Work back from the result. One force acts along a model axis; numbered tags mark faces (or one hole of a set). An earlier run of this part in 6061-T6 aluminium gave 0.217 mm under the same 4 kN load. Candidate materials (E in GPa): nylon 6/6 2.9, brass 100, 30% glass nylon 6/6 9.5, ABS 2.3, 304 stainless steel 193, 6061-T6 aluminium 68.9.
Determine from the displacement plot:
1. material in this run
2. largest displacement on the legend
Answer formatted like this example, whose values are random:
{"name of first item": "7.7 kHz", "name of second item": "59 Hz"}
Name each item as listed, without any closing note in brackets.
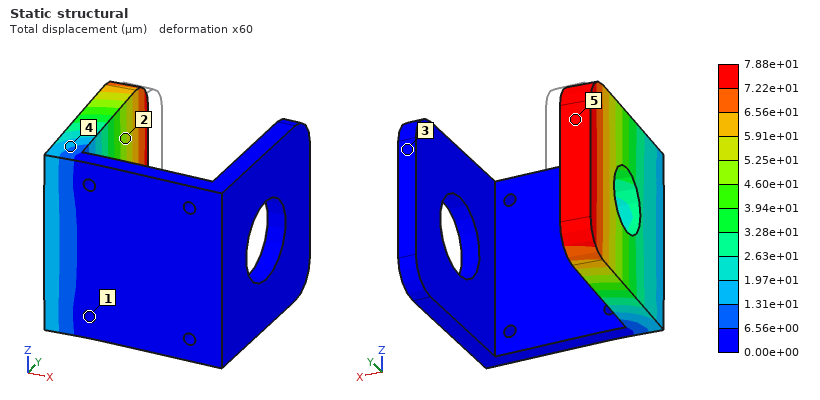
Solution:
{"material in this run": "304 stainless steel", "largest displacement on the legend": "7.88e+01 µm"}
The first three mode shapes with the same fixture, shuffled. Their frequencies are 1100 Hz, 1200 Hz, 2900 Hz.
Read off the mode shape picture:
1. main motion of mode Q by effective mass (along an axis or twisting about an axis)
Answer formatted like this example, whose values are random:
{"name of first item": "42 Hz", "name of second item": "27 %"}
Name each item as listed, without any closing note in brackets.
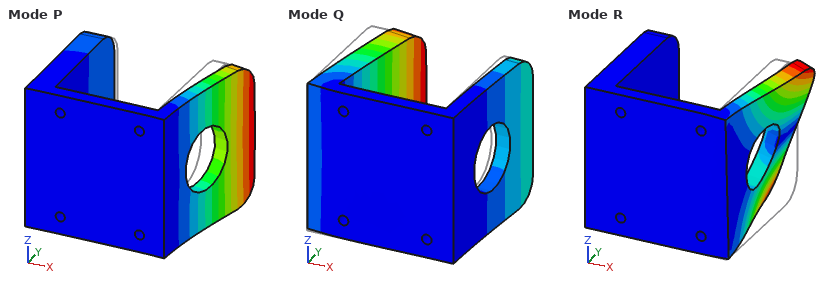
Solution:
{"main motion of mode Q by effective mass": "along X"}
